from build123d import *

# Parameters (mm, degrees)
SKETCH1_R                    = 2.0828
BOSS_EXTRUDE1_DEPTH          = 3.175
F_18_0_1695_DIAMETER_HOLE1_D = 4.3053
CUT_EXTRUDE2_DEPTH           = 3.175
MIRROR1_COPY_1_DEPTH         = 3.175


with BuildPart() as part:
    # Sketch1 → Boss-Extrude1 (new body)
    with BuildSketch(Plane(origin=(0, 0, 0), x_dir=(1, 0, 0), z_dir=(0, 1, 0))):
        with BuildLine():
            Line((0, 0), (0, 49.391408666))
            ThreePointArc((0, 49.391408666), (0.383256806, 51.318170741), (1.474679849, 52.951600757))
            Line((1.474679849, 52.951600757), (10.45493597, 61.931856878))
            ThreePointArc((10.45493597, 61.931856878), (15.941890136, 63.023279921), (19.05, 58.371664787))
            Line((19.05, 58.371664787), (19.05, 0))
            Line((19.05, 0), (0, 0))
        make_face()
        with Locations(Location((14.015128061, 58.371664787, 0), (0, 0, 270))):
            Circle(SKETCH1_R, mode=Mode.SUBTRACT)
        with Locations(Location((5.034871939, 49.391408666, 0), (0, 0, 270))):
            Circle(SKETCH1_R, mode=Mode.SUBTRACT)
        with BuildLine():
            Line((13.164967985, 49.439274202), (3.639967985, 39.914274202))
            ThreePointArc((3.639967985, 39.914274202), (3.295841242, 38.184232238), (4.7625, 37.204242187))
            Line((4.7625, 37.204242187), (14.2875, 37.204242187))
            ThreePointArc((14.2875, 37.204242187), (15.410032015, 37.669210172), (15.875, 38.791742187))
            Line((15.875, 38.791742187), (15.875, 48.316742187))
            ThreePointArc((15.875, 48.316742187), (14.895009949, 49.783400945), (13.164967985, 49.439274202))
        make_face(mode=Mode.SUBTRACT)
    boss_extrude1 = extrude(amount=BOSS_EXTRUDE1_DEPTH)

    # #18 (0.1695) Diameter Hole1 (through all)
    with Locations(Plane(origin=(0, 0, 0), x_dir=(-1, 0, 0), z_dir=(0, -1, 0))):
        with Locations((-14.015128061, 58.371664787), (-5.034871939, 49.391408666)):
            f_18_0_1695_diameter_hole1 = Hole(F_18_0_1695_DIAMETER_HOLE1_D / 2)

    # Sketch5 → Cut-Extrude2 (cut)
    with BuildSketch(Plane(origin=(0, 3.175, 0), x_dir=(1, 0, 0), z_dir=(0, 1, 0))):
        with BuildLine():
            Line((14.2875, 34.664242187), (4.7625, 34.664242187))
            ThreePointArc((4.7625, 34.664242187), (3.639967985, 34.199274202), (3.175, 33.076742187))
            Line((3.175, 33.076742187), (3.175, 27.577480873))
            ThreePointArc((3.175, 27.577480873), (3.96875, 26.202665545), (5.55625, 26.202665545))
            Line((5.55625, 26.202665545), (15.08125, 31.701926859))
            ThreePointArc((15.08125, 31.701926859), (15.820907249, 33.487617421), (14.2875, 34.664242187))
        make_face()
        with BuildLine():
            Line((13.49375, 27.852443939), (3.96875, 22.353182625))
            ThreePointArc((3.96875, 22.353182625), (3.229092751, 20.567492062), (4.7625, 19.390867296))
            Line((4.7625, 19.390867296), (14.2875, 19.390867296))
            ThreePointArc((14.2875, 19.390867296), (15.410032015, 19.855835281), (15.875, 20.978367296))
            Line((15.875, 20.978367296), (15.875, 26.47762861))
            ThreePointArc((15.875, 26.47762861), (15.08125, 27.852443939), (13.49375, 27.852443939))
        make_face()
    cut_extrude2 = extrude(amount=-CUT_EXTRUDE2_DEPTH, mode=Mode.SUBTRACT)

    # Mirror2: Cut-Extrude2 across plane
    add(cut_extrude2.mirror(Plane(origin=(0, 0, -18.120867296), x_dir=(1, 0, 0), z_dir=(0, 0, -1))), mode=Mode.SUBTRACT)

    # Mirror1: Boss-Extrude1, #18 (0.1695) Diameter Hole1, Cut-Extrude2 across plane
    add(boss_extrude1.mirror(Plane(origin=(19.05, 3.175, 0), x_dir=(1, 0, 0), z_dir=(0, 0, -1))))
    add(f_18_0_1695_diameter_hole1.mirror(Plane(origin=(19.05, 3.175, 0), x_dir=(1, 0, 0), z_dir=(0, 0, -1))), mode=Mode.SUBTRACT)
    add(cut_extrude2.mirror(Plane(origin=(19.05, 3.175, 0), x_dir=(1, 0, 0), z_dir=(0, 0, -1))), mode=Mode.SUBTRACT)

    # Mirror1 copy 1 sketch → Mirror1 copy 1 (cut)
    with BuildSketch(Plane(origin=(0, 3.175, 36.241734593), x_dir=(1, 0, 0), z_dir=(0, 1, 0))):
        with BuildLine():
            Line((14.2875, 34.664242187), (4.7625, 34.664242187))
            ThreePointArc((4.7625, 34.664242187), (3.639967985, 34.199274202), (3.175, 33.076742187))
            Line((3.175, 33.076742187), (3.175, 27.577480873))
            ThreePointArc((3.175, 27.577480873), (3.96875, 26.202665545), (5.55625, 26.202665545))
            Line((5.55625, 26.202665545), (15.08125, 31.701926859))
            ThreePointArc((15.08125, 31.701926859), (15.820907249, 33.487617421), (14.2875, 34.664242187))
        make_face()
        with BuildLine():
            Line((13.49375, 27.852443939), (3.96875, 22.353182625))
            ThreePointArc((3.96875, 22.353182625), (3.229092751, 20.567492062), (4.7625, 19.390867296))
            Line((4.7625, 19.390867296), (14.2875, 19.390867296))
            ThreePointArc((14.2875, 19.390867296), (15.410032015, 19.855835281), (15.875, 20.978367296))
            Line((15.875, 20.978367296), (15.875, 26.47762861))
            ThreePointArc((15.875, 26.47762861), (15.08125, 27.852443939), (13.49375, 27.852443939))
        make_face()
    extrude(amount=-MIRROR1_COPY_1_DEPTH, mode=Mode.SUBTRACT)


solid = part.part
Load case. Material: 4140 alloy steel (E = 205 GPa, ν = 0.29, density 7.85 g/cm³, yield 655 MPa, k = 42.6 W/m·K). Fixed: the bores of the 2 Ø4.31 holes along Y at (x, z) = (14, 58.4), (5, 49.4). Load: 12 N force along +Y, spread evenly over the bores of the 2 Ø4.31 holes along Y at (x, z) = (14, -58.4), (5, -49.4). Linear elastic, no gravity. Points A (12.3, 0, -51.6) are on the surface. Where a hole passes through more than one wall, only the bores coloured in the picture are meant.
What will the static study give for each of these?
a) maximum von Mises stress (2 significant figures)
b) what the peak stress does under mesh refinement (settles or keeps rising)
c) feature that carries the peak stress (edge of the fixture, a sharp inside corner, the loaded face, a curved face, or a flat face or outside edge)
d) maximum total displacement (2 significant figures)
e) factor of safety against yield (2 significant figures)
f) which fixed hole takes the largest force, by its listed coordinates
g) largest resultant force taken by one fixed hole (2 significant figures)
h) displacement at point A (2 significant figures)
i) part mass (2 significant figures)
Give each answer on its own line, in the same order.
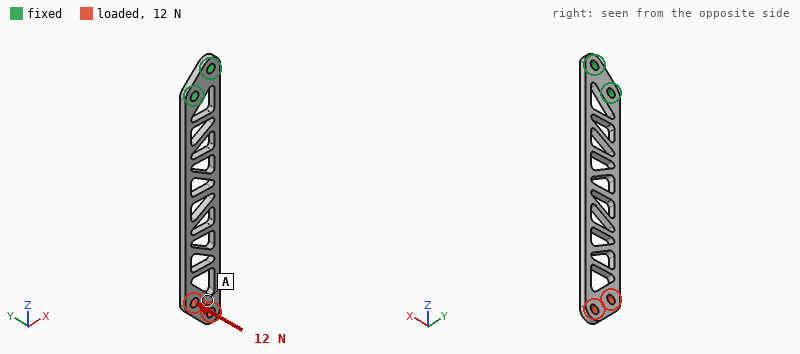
190 MPa
settles
a curved face
1.3 mm
3.5
(5, 49.4)
38 N
1.1 mm
35 g
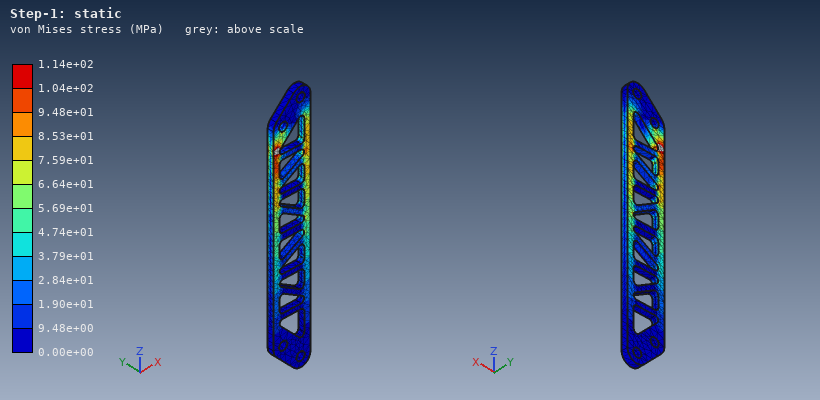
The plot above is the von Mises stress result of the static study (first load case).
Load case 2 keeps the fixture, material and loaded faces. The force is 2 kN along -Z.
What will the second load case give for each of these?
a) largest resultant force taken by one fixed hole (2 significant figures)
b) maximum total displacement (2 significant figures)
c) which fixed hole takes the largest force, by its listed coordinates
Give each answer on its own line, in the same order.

1.1 kN
57 µm
(5, 49.4)
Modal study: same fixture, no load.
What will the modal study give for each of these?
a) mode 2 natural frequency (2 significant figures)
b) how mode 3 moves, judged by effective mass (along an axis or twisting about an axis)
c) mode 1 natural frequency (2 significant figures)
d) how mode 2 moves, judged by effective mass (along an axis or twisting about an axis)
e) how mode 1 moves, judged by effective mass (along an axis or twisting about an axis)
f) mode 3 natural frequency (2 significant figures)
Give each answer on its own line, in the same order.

1100 Hz
along X
170 Hz
along Y
along Y
1100 Hz
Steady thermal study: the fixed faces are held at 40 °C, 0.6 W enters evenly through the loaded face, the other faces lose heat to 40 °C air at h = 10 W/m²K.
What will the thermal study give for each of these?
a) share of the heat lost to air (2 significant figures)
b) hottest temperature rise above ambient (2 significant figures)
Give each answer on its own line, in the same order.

78 %
25 K
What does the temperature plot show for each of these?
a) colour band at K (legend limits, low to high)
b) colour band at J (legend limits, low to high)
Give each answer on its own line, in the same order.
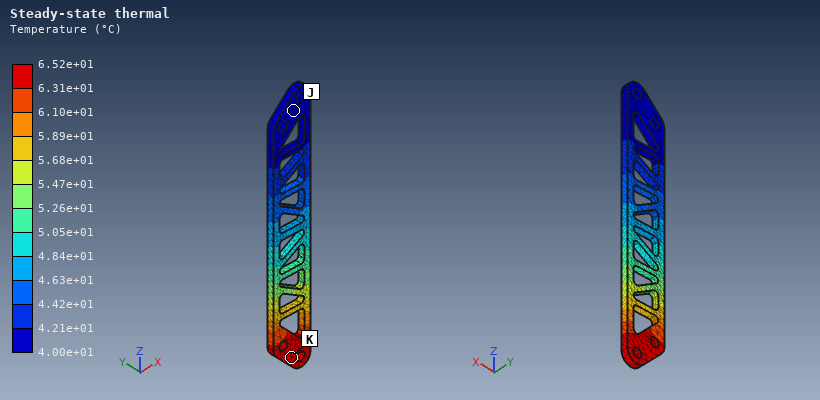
6.31e+01 to 6.52e+01 °C
4.00e+01 to 4.21e+01 °C
